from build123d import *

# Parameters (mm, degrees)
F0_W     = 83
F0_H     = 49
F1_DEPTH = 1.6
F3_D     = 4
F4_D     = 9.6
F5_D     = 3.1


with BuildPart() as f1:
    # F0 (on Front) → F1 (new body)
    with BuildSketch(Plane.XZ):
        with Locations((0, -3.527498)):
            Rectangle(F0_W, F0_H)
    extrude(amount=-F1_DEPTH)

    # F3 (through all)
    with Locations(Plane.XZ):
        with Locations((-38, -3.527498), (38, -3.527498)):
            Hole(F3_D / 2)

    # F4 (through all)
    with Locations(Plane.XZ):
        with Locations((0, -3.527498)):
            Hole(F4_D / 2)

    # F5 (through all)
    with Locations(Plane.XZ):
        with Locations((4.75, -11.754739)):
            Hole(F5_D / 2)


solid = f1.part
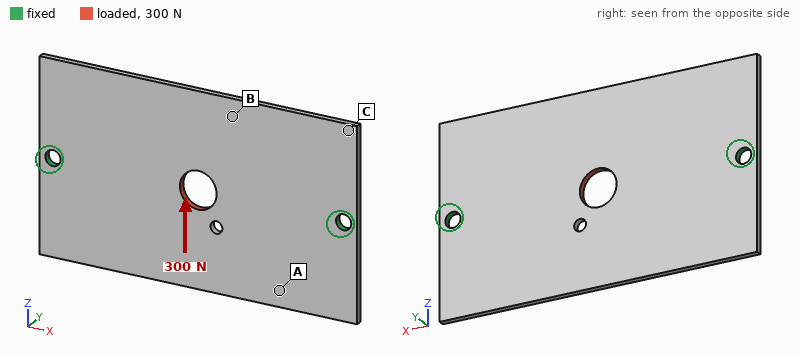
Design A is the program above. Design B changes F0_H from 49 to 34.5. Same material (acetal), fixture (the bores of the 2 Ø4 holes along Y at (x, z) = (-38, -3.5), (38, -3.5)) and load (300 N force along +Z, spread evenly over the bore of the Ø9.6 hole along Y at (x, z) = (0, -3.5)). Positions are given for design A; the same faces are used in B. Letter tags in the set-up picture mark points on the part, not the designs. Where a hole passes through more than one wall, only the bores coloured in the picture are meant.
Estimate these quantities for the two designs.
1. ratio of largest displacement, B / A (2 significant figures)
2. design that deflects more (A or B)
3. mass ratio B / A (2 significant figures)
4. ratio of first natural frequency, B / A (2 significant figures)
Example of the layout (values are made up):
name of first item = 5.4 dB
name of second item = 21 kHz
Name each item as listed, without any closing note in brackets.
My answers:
ratio of largest displacement, B / A = 1.8
design that deflects more = B
mass ratio B / A = 0.70
ratio of first natural frequency, B / A = 1.3
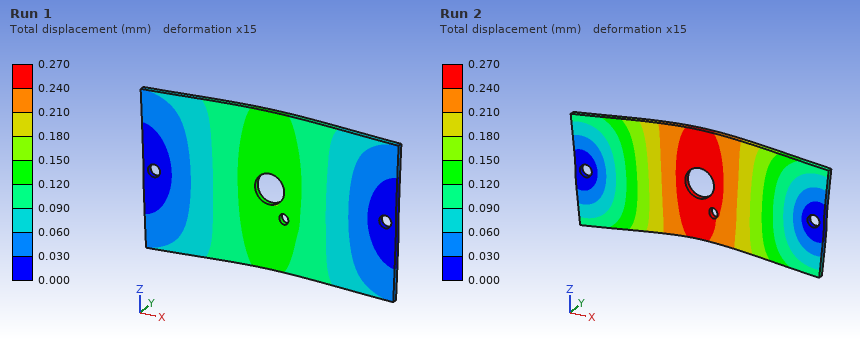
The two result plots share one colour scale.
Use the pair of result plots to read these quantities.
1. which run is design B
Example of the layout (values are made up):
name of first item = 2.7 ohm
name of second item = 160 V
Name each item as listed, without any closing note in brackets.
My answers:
which run is design B = Run 2
